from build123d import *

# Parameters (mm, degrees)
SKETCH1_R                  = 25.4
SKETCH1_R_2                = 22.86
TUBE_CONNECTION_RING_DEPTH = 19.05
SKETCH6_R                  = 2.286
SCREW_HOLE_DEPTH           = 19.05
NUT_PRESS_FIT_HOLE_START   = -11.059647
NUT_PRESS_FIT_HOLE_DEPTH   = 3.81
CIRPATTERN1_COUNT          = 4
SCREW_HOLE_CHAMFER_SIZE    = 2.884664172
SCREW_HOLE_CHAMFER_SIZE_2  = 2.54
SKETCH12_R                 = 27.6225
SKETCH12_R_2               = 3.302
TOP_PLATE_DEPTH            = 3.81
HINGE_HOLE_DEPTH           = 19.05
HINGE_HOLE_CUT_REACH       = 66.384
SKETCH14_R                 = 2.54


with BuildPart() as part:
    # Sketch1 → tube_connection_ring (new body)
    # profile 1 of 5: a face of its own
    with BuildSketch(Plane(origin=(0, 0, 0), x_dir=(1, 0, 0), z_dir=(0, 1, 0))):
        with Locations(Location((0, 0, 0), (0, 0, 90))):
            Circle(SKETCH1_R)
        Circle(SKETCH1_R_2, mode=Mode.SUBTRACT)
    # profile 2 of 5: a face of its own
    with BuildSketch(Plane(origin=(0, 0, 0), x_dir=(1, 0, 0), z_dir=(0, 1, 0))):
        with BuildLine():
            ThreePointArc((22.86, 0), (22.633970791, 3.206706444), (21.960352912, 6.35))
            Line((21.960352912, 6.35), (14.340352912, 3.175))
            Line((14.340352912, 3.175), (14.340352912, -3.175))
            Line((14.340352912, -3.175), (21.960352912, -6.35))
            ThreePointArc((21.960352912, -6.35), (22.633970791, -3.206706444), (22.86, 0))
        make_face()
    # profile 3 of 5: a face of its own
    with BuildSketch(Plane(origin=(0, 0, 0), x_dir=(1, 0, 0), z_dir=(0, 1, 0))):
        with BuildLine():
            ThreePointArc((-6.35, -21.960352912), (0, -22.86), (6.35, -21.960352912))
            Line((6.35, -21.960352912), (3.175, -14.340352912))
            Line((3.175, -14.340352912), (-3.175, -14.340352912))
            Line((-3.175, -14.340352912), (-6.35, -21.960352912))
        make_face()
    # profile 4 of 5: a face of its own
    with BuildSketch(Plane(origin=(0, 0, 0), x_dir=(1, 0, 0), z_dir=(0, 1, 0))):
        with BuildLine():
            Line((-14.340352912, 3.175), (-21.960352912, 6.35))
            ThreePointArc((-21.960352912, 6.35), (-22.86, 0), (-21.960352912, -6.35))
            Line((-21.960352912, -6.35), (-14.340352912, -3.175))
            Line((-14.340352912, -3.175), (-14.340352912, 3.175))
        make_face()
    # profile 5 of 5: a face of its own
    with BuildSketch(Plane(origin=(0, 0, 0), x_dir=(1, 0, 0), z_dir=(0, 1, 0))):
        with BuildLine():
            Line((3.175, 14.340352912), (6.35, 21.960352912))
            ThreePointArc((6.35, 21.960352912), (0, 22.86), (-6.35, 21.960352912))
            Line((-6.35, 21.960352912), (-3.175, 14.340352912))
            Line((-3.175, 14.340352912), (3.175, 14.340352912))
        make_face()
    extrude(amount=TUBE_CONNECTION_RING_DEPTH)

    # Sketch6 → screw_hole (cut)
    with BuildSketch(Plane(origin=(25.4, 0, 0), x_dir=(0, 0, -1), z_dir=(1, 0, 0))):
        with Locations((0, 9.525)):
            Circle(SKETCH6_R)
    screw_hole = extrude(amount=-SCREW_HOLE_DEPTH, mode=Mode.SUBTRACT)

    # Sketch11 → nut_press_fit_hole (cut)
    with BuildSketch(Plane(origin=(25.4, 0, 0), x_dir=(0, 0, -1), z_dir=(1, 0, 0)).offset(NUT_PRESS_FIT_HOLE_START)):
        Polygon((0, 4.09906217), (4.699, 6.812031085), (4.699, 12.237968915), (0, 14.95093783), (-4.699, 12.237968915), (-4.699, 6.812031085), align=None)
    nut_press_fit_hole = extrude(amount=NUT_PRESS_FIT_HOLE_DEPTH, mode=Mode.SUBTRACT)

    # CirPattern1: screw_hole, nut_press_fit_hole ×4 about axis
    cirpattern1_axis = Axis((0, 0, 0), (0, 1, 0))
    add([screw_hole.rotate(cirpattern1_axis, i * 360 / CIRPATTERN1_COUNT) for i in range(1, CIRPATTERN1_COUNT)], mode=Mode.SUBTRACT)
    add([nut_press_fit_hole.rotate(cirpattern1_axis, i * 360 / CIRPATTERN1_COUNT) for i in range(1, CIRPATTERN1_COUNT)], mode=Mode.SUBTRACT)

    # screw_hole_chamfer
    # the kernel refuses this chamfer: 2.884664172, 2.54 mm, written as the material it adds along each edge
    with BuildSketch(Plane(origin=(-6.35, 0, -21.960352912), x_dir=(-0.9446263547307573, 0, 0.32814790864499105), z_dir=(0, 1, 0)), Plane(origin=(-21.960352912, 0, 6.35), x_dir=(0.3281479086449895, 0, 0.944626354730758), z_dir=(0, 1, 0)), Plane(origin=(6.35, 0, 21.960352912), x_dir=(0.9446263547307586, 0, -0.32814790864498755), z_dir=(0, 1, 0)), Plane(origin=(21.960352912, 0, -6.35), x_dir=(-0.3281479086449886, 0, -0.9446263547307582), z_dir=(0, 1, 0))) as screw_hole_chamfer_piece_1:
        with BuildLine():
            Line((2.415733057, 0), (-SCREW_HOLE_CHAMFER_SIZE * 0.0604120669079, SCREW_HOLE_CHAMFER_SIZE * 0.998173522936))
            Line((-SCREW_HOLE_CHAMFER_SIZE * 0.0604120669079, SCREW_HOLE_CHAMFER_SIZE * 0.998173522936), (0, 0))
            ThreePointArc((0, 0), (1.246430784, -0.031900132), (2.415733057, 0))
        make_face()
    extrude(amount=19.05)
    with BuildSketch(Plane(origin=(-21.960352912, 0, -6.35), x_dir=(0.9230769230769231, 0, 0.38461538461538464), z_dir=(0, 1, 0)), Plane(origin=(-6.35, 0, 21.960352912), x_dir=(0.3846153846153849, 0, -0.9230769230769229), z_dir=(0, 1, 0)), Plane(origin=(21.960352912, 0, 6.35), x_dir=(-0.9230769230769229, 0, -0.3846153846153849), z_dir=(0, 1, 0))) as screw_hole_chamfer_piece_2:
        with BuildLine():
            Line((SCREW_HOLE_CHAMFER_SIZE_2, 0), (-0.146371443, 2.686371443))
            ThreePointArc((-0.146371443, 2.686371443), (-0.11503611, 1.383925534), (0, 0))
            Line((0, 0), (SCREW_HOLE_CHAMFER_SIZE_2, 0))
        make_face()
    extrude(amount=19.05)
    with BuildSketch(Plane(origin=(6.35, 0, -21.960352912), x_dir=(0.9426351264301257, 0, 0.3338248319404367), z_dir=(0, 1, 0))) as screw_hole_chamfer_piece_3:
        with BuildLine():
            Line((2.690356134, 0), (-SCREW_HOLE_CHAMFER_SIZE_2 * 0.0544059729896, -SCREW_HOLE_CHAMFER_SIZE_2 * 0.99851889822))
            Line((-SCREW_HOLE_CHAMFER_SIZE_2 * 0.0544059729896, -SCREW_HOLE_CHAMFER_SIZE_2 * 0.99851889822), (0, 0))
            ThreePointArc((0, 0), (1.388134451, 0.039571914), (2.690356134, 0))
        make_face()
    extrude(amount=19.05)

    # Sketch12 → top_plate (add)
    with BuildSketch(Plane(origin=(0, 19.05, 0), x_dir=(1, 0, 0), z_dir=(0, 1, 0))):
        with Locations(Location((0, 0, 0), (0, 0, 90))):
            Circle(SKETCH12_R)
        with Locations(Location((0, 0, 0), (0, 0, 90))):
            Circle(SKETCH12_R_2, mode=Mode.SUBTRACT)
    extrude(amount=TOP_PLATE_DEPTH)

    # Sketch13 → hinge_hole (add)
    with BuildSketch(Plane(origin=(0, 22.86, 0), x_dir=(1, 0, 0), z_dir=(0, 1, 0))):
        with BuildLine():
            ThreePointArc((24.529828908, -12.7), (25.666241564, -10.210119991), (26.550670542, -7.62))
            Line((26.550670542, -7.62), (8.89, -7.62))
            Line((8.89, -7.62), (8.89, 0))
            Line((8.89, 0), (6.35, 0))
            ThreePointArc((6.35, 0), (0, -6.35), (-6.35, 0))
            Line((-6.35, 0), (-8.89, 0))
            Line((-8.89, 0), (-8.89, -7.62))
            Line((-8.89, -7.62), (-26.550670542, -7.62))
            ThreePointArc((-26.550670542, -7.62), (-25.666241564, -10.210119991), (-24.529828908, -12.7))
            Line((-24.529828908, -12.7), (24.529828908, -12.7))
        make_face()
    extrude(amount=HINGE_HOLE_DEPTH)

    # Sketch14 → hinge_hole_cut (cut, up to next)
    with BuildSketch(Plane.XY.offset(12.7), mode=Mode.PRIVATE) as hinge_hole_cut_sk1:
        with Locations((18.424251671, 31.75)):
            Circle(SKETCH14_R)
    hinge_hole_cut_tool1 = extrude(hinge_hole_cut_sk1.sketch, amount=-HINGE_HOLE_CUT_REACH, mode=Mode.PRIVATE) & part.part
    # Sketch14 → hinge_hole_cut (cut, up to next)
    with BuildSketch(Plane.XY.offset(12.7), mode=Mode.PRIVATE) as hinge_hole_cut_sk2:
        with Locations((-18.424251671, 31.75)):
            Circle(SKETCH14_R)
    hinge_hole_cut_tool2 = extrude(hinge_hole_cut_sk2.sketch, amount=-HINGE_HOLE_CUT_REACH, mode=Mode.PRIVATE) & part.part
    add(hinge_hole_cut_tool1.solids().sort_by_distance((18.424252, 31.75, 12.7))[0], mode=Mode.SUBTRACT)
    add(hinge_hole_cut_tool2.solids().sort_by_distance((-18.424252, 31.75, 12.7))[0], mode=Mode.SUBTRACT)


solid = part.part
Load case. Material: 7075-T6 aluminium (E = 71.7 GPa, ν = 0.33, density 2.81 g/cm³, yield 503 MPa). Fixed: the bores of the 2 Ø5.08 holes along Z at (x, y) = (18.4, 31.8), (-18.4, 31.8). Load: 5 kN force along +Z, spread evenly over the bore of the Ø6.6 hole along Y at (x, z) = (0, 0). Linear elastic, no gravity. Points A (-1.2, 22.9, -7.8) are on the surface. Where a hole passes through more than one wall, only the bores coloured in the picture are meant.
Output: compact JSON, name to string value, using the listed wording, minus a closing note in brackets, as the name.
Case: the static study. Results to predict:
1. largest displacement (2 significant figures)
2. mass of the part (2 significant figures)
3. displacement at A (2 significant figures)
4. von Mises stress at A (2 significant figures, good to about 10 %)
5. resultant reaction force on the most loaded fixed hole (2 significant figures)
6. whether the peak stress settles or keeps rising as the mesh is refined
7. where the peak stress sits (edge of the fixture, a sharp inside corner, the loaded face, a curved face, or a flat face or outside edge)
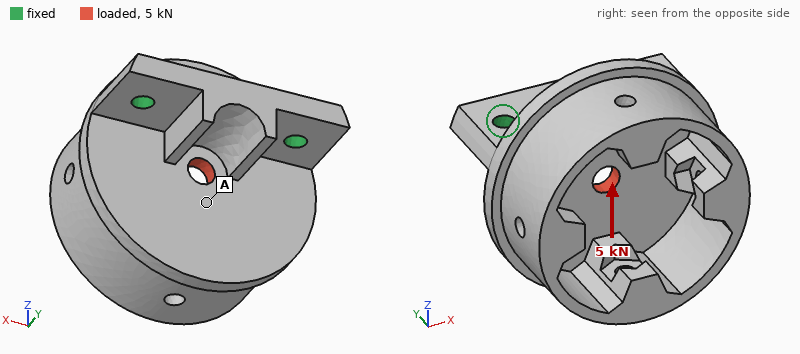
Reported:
{"largest displacement": "0.27 mm", "mass of the part": "78 g", "displacement at A": "0.12 mm", "von Mises stress at A": "39 MPa", "resultant reaction force on the most loaded fixed hole": "2.5 kN", "whether the peak stress settles or keeps rising as the mesh is refined": "keeps rising", "where the peak stress sits": "edge of the fixture"}
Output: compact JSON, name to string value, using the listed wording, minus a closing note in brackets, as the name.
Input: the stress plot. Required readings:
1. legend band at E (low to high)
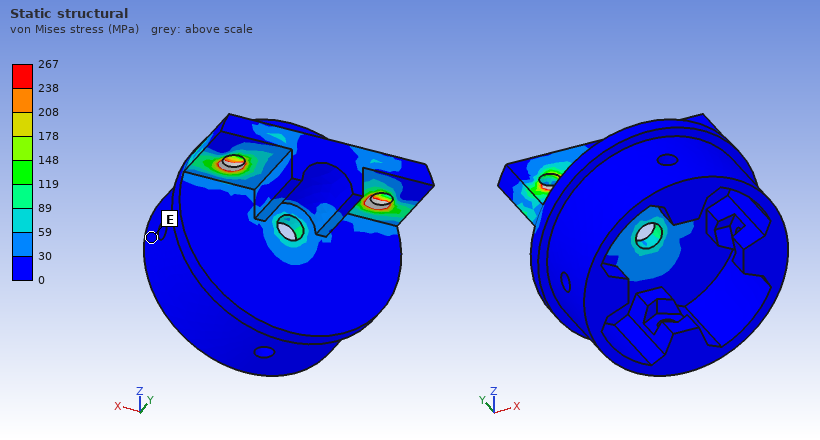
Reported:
{"legend band at E": "0 to 30 MPa"}
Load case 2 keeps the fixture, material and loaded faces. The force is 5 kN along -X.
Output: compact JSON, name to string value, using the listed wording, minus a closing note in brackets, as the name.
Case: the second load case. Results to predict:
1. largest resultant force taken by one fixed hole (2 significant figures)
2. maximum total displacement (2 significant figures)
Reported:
{"largest resultant force taken by one fixed hole": "3.1 kN", "maximum total displacement": "48 µm"}
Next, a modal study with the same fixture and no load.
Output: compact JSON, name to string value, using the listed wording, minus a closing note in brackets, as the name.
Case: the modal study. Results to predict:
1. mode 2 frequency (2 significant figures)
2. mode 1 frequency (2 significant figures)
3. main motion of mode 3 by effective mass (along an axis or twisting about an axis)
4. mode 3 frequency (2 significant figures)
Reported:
{"mode 2 frequency": "5800 Hz", "mode 1 frequency": "1900 Hz", "main motion of mode 3 by effective mass": "along X", "mode 3 frequency": "6100 Hz"}
